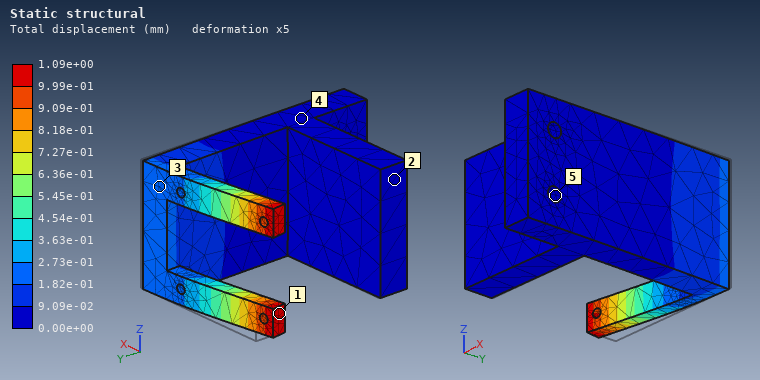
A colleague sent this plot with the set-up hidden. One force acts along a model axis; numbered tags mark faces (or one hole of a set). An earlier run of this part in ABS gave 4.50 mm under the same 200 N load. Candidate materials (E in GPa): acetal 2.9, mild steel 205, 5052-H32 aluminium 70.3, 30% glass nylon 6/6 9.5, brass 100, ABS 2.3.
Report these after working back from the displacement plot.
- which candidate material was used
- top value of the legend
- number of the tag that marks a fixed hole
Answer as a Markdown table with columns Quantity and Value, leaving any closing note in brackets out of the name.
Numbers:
| Quantity | Value |
|---|---|
| which candidate material was used | 30% glass nylon 6/6 |
| top value of the legend | 1.09e+00 mm |
| number of the tag that marks a fixed hole | 5 |
